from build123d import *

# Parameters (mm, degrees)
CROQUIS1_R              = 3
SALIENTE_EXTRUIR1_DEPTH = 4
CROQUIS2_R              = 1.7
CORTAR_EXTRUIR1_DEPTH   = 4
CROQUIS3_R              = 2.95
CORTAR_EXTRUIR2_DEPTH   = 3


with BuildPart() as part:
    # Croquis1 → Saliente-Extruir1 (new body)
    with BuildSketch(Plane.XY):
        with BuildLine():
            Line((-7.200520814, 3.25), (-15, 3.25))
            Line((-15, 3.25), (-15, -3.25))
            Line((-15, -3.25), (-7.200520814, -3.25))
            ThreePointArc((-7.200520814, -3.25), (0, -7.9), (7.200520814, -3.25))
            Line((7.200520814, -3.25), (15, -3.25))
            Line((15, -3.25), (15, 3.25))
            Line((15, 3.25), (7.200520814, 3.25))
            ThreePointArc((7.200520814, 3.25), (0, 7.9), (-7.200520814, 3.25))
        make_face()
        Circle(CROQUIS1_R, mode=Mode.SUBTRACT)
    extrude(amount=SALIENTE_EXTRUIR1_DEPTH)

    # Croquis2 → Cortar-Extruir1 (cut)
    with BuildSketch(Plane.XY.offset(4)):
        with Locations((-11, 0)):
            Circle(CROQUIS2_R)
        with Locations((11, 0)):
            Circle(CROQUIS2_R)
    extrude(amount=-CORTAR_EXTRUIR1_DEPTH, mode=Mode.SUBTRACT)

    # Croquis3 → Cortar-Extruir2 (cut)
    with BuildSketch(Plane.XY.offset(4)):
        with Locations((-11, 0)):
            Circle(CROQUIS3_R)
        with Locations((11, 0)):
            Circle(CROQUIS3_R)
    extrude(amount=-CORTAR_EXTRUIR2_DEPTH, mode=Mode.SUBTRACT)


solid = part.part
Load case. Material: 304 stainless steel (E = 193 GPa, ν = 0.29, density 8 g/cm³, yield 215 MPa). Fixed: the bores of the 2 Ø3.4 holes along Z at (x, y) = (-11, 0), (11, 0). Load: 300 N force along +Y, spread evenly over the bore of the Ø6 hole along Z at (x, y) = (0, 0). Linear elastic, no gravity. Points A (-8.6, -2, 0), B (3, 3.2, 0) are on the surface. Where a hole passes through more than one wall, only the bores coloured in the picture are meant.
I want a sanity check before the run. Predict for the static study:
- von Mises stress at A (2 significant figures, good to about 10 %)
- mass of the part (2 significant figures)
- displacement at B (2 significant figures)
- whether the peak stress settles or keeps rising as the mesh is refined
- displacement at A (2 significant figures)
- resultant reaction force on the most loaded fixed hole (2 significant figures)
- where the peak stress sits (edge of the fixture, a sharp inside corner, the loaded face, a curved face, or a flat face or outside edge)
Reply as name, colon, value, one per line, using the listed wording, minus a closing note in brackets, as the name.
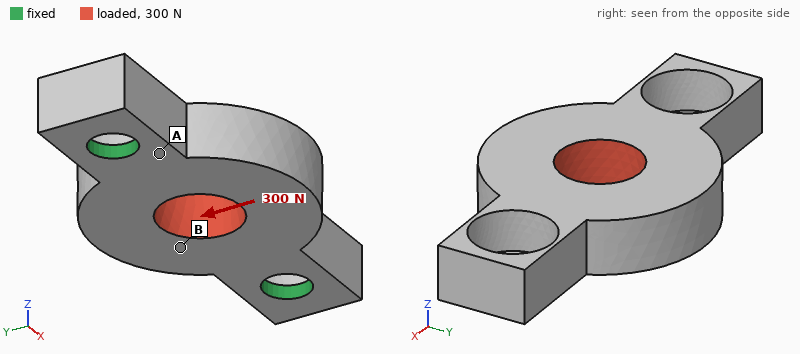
von Mises stress at A: 25 MPa
mass of the part: 7.0 g
displacement at B: 1.9 µm
whether the peak stress settles or keeps rising as the mesh is refined: keeps rising
displacement at A: 0.80 µm
resultant reaction force on the most loaded fixed hole: 150 N
where the peak stress sits: edge of the fixture
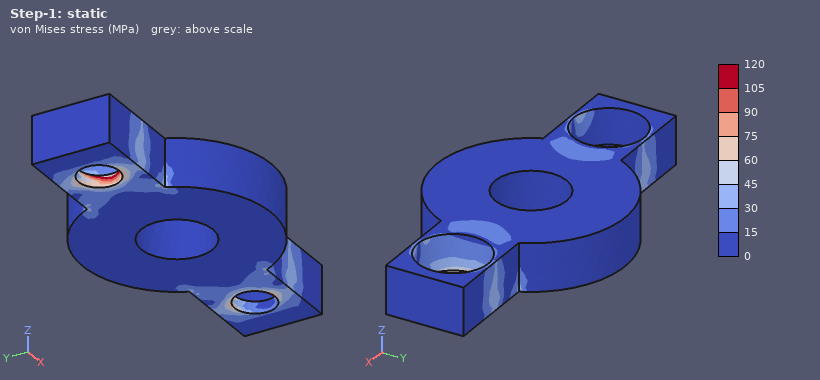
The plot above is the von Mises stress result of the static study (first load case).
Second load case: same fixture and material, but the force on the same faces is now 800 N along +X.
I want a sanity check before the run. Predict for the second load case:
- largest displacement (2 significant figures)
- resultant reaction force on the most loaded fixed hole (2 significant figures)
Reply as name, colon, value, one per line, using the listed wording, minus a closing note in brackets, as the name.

largest displacement: 1.5 µm
resultant reaction force on the most loaded fixed hole: 400 N
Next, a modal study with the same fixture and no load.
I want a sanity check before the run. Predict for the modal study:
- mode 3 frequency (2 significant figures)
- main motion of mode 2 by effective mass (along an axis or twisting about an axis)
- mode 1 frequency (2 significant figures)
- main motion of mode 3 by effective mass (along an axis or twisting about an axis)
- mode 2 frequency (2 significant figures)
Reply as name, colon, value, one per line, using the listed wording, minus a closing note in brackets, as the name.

mode 3 frequency: 36 kHz
main motion of mode 2 by effective mass: along Z
mode 1 frequency: 13 kHz
main motion of mode 3 by effective mass: along Y
mode 2 frequency: 20 kHz
